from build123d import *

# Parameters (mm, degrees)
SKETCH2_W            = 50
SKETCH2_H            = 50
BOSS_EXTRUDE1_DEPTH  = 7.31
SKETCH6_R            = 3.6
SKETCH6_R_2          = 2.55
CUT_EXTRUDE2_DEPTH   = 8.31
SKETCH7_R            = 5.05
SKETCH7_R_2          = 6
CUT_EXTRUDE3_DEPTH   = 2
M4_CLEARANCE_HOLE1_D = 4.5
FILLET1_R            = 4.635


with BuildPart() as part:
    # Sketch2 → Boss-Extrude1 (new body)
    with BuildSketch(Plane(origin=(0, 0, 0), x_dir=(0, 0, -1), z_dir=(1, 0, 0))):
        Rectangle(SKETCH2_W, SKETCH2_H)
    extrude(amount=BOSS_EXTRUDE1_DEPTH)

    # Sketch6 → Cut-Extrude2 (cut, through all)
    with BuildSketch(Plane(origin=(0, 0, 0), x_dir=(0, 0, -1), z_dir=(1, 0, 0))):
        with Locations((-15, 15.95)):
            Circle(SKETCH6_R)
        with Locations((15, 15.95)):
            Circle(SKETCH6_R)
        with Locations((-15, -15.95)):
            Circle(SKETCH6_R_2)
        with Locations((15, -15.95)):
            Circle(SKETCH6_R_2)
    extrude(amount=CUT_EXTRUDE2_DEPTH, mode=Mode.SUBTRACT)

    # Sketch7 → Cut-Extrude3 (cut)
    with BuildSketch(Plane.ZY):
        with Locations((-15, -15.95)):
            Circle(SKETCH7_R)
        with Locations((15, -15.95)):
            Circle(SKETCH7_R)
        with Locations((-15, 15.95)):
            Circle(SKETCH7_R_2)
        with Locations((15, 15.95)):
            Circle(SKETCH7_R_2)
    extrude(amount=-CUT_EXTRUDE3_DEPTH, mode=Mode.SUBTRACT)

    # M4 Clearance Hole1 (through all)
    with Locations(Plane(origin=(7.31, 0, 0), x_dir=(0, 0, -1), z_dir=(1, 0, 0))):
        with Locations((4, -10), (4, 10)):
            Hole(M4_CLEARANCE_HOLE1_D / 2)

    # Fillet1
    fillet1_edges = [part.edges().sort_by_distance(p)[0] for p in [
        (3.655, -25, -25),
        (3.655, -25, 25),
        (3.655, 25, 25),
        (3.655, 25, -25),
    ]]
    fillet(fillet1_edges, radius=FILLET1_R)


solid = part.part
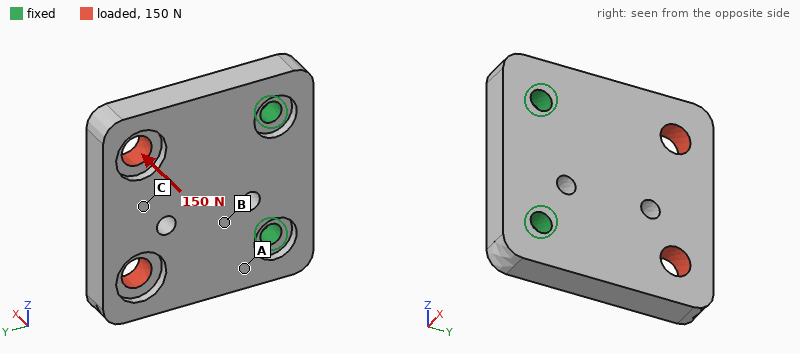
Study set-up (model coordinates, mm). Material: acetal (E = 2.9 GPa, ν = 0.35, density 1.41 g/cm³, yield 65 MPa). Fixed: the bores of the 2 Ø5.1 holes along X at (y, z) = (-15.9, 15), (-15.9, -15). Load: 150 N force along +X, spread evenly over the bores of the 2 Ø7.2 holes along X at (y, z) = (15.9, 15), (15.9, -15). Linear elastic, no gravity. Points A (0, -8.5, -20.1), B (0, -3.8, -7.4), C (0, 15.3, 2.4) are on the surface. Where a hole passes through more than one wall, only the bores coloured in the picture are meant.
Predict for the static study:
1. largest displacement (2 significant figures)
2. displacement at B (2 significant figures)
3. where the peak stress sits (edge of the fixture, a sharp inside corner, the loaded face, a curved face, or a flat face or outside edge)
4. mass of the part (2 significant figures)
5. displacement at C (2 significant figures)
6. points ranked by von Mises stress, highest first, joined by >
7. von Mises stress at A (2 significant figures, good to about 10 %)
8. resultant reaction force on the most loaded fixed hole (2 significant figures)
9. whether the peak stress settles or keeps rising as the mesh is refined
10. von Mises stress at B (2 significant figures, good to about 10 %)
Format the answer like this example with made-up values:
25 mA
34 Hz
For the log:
0.74 mm
0.16 mm
edge of the fixture
23 g
0.52 mm
A > B > C
9.3 MPa
77 N
keeps rising
5.6 MPa
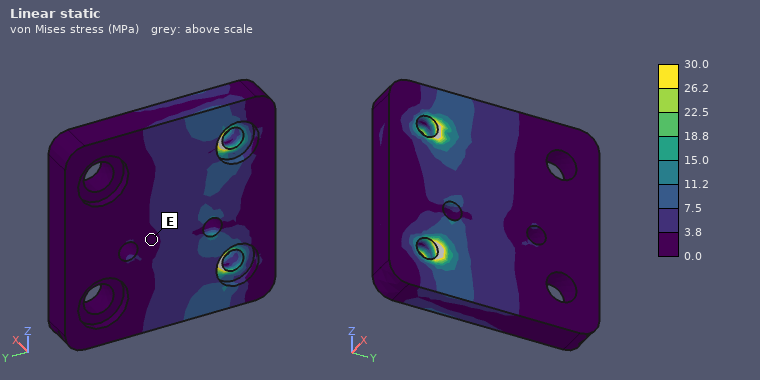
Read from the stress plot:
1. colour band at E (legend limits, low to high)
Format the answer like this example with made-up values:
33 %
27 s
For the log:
0.0 to 3.8 MPa
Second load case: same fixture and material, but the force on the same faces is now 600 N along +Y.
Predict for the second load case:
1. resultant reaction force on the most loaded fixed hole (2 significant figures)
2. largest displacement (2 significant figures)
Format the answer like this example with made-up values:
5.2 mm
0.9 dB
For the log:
300 N
93 µm
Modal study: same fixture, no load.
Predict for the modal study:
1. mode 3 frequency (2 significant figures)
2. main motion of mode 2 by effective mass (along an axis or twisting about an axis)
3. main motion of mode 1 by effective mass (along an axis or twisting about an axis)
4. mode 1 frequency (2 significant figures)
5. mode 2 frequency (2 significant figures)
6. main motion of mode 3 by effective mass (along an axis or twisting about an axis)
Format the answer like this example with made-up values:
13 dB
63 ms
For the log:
3400 Hz
twisting about Y
along X
870 Hz
1900 Hz
along Z
